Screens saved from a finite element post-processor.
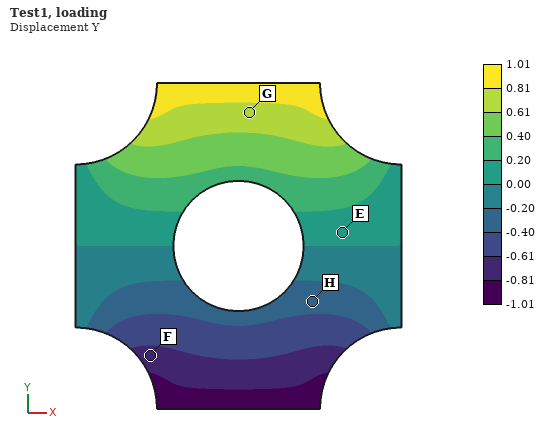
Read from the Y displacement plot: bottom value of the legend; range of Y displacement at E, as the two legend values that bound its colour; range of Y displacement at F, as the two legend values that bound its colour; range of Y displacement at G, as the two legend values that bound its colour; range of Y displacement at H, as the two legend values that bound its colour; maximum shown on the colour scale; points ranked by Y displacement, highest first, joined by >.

-1.01
0.00 to 0.20
-0.81 to -0.61
0.61 to 0.81
-0.40 to -0.20
1.01
G > E > H > F
